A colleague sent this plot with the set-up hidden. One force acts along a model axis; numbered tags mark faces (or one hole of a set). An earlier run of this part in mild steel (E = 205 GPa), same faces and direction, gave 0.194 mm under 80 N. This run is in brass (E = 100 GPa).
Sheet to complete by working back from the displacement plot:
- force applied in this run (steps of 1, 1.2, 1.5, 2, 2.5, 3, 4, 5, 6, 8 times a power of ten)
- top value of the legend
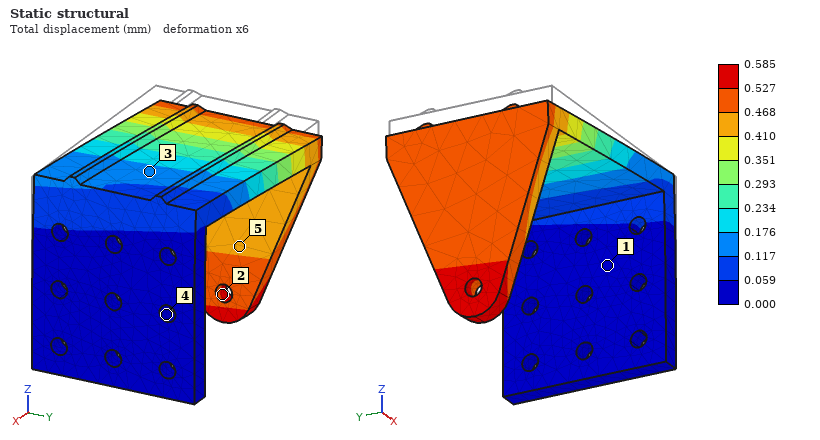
120 N
0.585 mm
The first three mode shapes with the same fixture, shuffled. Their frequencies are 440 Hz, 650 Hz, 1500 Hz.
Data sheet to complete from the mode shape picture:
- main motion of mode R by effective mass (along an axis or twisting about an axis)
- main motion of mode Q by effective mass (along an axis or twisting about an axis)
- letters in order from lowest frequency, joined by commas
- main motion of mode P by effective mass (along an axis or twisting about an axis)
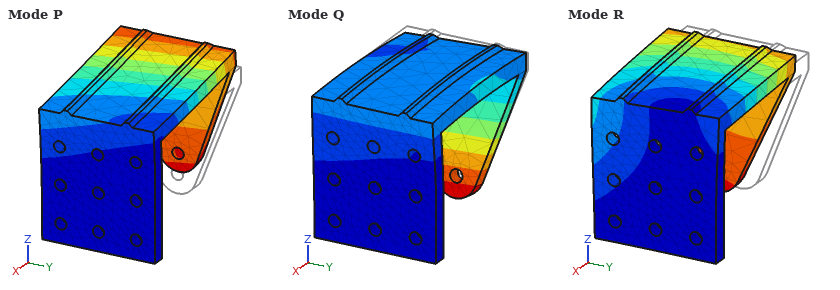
along Y
along X
P, R, Q
along Z
